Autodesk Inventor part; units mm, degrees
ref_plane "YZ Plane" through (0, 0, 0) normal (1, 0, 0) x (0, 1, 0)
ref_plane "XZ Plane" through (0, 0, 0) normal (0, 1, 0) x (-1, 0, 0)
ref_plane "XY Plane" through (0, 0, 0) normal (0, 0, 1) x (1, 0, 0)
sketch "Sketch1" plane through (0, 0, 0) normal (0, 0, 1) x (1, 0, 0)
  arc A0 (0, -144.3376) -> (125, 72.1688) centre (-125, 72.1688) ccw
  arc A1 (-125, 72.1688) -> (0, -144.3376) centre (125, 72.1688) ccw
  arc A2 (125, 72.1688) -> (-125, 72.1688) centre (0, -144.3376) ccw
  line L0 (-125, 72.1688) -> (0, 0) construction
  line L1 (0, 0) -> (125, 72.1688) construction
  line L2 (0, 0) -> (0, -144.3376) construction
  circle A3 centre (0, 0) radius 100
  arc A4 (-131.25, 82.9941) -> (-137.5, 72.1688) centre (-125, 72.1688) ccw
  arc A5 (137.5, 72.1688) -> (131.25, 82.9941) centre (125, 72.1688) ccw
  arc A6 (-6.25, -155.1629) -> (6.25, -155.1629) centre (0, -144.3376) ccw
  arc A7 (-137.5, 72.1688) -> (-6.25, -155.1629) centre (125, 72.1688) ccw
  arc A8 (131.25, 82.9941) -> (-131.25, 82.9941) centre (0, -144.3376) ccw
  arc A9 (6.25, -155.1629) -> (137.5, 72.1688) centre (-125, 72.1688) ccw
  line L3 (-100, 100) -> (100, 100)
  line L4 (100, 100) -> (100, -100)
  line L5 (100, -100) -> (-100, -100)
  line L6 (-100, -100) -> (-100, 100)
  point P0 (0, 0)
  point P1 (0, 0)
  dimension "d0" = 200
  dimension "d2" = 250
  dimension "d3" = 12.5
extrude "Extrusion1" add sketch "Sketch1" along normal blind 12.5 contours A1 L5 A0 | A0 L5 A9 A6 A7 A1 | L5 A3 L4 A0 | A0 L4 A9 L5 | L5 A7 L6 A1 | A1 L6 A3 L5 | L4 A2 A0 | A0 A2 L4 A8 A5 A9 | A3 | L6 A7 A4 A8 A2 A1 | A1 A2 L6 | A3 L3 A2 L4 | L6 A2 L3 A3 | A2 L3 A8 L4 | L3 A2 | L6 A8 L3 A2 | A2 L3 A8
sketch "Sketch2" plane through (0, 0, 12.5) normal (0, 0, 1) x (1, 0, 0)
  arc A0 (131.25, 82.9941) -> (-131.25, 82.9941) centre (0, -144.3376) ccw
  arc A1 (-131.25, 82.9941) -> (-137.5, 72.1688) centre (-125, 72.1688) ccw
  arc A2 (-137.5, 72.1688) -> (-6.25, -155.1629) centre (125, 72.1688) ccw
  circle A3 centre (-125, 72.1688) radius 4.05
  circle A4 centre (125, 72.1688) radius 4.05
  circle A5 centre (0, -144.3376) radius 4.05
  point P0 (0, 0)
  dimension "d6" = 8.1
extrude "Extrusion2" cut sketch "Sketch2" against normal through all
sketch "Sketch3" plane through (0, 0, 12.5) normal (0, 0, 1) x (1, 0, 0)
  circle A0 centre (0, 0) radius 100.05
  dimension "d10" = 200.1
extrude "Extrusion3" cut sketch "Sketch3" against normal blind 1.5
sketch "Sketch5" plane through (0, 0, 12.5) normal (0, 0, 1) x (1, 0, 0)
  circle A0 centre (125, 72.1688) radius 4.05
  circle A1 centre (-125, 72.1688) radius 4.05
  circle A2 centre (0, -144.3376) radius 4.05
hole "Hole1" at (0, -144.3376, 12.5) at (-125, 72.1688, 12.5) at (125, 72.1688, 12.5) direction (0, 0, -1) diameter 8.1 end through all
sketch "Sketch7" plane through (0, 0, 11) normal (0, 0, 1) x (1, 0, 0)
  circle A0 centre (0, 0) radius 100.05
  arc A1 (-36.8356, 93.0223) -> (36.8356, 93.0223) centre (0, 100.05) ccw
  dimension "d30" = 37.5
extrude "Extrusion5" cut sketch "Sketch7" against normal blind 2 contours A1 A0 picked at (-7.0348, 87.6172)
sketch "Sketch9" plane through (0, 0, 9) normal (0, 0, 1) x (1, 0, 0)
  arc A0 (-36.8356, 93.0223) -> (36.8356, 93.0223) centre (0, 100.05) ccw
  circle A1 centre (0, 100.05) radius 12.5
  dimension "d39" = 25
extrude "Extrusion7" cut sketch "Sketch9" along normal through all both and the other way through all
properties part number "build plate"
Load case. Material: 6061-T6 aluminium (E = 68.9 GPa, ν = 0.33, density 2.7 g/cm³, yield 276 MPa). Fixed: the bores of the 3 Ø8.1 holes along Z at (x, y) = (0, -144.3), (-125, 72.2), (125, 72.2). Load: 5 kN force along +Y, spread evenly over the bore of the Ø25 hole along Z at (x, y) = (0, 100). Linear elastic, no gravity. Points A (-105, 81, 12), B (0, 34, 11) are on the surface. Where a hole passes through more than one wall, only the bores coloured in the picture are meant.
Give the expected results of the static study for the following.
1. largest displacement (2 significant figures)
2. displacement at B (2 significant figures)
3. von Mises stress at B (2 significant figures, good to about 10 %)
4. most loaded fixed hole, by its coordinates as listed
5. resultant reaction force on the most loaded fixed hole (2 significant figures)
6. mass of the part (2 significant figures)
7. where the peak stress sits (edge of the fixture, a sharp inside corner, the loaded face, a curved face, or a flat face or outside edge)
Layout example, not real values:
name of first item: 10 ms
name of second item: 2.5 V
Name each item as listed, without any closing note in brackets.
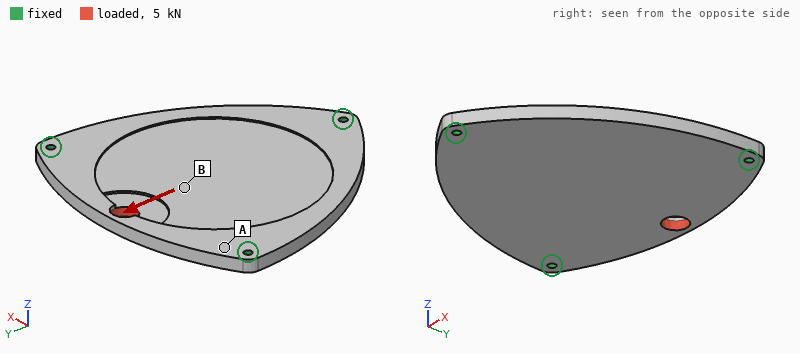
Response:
largest displacement: 25 µm
displacement at B: 7.5 µm
von Mises stress at B: 3.3 MPa
most loaded fixed hole, by its coordinates as listed: (0, -144.3)
resultant reaction force on the most loaded fixed hole: 2.0 kN
mass of the part: 1.7 kg
where the peak stress sits: a curved face
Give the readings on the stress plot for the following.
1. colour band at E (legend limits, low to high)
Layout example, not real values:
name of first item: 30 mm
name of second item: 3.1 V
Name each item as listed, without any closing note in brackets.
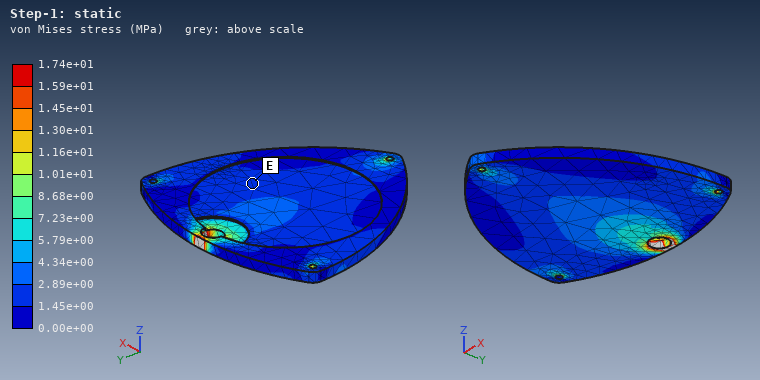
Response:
colour band at E: 1.45e+00 to 2.89e+00 MPa
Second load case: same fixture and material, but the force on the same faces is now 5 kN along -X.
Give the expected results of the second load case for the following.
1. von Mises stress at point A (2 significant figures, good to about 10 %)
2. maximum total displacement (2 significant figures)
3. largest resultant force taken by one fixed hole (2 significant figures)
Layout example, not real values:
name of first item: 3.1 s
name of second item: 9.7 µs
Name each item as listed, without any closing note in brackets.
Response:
von Mises stress at point A: 6.4 MPa
maximum total displacement: 12 µm
largest resultant force taken by one fixed hole: 2.5 kN
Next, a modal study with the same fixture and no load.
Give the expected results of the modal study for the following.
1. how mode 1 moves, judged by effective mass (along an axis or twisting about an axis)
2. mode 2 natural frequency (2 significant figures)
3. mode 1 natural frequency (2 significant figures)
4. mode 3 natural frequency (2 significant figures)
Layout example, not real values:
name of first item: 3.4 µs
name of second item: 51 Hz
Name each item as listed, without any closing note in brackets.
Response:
how mode 1 moves, judged by effective mass: along Z
mode 2 natural frequency: 960 Hz
mode 1 natural frequency: 740 Hz
mode 3 natural frequency: 980 Hz
